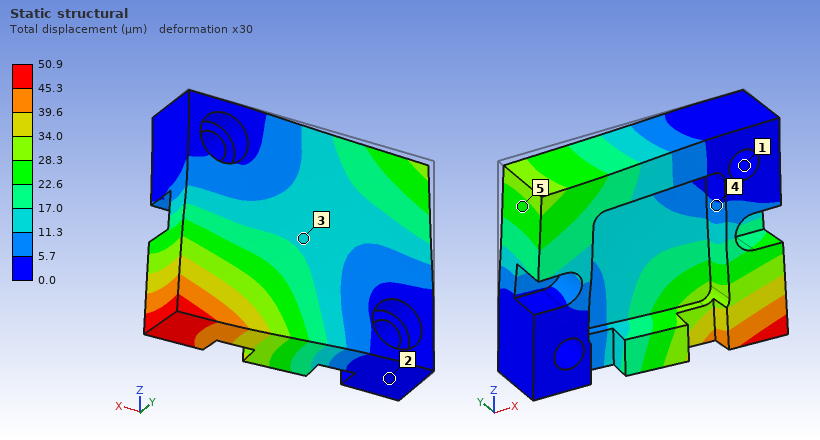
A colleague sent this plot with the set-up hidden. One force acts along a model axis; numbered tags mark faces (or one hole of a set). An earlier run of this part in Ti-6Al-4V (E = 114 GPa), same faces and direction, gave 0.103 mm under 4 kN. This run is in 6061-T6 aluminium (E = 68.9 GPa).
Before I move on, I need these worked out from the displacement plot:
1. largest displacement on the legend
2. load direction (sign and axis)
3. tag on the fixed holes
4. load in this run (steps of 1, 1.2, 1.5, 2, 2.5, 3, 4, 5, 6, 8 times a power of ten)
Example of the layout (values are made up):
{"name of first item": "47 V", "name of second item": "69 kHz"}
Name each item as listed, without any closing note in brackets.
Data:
{"largest displacement on the legend": "50.9 µm", "load direction": "-Y", "tag on the fixed holes": "1", "load in this run": "1.2 kN"}
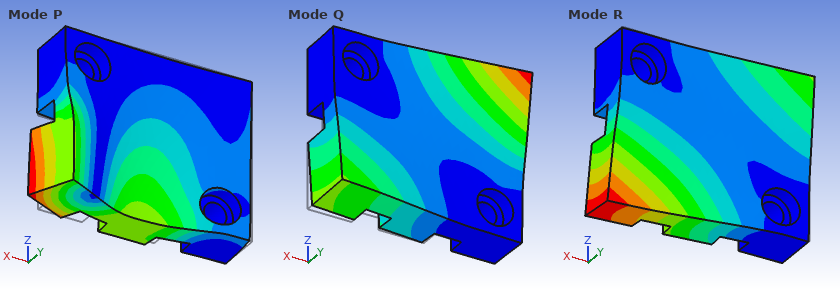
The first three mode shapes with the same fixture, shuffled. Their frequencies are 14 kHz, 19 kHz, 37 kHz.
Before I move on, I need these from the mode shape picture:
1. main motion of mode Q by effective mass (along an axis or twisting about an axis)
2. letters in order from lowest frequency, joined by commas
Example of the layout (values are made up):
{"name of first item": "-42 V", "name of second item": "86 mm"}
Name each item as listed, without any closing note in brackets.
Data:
{"main motion of mode Q by effective mass": "along Y", "letters in order from lowest frequency, joined by commas": "R, Q, P"}
